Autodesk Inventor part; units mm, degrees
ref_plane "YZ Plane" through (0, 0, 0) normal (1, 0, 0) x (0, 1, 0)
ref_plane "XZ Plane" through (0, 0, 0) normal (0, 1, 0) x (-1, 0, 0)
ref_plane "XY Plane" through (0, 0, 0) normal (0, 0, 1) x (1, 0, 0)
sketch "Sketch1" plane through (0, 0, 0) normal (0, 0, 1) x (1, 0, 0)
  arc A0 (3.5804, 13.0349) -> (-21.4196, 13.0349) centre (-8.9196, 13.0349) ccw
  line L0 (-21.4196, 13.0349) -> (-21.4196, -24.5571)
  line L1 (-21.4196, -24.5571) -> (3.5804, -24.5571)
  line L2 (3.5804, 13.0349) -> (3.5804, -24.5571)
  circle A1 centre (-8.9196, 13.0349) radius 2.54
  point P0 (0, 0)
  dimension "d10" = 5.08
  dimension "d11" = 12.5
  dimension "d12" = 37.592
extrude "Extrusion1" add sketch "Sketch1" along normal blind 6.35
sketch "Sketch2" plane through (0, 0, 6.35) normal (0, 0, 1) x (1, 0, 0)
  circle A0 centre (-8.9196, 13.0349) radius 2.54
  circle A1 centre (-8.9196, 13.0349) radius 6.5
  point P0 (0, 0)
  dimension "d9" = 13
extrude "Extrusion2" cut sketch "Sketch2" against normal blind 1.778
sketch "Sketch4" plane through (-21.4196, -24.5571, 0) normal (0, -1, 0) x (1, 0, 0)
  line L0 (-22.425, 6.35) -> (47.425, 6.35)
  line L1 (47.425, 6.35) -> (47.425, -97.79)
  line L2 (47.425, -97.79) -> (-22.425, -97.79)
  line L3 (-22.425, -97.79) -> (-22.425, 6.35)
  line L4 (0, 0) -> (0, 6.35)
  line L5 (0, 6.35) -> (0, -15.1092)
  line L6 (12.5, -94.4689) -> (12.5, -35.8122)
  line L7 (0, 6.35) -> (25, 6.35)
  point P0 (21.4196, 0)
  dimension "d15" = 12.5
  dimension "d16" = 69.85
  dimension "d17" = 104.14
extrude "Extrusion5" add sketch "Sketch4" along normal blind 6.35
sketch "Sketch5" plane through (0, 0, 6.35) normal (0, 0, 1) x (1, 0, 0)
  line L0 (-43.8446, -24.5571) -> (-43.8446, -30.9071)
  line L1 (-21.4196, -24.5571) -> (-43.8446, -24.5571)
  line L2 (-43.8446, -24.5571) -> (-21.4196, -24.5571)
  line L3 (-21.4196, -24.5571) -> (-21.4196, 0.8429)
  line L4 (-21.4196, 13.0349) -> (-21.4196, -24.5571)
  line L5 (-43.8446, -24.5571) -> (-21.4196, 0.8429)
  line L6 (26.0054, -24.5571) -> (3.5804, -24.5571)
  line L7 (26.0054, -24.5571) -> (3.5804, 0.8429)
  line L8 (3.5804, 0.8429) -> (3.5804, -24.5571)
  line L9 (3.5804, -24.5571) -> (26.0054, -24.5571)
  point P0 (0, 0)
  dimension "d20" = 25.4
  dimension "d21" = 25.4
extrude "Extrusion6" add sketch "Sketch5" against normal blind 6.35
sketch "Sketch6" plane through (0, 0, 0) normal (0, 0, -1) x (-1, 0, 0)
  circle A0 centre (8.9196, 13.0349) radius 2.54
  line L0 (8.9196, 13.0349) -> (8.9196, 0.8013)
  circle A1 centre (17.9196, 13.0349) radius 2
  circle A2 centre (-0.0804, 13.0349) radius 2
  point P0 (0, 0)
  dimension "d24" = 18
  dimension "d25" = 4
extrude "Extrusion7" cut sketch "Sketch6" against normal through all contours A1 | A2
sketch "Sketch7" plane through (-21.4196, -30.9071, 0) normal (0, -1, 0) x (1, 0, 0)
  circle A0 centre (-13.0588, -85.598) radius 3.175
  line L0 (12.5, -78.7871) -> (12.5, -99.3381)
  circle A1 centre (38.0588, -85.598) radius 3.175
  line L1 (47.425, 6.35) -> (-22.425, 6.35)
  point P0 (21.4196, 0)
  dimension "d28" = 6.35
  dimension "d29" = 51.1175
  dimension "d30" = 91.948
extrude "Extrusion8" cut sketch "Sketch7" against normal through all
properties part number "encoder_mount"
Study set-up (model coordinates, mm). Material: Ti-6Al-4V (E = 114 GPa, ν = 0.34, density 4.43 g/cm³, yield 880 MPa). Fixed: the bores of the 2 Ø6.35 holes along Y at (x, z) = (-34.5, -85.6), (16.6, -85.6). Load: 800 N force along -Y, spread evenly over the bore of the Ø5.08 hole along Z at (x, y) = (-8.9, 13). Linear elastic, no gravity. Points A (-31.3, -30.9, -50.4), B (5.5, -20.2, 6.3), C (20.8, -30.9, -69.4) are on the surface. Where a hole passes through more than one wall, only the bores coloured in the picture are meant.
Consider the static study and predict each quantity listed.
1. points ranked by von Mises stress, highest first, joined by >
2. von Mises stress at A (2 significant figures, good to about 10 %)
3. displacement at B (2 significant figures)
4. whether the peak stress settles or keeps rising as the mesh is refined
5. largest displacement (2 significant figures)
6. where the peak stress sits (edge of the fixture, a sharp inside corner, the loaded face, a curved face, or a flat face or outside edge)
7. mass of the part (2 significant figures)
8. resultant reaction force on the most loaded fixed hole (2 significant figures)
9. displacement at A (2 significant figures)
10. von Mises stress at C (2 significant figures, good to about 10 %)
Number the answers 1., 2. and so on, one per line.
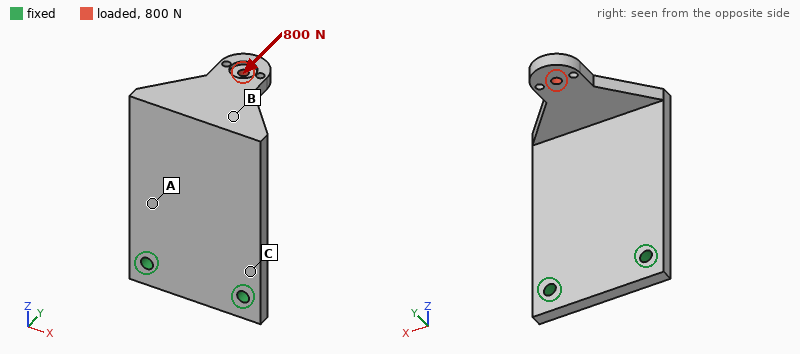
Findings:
1. C > A > B
2. 88 MPa
3. 1.2 mm
4. keeps rising
5. 1.5 mm
6. edge of the fixture
7. 250 g
8. 400 N
9. 0.25 mm
10. 130 MPa
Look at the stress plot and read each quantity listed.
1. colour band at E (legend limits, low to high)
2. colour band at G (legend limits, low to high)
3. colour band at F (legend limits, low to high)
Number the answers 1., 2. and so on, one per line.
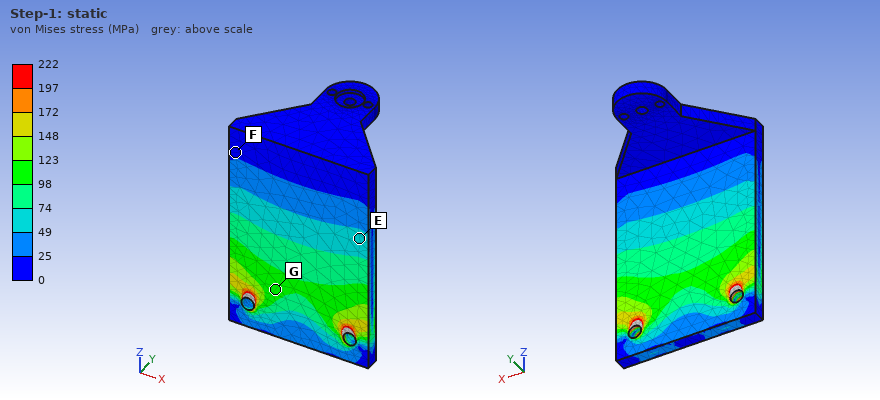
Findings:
1. 49 to 74 MPa
2. 98 to 123 MPa
3. 0 to 25 MPa
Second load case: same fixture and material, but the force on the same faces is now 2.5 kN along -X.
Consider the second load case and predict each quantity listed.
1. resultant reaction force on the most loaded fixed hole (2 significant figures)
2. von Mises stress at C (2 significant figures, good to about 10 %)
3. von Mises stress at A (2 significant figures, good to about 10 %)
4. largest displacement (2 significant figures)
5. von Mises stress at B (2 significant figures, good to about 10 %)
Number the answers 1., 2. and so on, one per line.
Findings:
1. 4.7 kN
2. 170 MPa
3. 160 MPa
4. 1.5 mm
5. 88 MPa
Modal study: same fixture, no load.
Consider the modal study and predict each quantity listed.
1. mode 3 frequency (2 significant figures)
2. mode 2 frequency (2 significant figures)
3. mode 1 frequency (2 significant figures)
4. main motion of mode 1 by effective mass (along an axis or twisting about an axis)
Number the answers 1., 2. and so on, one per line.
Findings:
1. 1800 Hz
2. 1200 Hz
3. 410 Hz
4. along Y
